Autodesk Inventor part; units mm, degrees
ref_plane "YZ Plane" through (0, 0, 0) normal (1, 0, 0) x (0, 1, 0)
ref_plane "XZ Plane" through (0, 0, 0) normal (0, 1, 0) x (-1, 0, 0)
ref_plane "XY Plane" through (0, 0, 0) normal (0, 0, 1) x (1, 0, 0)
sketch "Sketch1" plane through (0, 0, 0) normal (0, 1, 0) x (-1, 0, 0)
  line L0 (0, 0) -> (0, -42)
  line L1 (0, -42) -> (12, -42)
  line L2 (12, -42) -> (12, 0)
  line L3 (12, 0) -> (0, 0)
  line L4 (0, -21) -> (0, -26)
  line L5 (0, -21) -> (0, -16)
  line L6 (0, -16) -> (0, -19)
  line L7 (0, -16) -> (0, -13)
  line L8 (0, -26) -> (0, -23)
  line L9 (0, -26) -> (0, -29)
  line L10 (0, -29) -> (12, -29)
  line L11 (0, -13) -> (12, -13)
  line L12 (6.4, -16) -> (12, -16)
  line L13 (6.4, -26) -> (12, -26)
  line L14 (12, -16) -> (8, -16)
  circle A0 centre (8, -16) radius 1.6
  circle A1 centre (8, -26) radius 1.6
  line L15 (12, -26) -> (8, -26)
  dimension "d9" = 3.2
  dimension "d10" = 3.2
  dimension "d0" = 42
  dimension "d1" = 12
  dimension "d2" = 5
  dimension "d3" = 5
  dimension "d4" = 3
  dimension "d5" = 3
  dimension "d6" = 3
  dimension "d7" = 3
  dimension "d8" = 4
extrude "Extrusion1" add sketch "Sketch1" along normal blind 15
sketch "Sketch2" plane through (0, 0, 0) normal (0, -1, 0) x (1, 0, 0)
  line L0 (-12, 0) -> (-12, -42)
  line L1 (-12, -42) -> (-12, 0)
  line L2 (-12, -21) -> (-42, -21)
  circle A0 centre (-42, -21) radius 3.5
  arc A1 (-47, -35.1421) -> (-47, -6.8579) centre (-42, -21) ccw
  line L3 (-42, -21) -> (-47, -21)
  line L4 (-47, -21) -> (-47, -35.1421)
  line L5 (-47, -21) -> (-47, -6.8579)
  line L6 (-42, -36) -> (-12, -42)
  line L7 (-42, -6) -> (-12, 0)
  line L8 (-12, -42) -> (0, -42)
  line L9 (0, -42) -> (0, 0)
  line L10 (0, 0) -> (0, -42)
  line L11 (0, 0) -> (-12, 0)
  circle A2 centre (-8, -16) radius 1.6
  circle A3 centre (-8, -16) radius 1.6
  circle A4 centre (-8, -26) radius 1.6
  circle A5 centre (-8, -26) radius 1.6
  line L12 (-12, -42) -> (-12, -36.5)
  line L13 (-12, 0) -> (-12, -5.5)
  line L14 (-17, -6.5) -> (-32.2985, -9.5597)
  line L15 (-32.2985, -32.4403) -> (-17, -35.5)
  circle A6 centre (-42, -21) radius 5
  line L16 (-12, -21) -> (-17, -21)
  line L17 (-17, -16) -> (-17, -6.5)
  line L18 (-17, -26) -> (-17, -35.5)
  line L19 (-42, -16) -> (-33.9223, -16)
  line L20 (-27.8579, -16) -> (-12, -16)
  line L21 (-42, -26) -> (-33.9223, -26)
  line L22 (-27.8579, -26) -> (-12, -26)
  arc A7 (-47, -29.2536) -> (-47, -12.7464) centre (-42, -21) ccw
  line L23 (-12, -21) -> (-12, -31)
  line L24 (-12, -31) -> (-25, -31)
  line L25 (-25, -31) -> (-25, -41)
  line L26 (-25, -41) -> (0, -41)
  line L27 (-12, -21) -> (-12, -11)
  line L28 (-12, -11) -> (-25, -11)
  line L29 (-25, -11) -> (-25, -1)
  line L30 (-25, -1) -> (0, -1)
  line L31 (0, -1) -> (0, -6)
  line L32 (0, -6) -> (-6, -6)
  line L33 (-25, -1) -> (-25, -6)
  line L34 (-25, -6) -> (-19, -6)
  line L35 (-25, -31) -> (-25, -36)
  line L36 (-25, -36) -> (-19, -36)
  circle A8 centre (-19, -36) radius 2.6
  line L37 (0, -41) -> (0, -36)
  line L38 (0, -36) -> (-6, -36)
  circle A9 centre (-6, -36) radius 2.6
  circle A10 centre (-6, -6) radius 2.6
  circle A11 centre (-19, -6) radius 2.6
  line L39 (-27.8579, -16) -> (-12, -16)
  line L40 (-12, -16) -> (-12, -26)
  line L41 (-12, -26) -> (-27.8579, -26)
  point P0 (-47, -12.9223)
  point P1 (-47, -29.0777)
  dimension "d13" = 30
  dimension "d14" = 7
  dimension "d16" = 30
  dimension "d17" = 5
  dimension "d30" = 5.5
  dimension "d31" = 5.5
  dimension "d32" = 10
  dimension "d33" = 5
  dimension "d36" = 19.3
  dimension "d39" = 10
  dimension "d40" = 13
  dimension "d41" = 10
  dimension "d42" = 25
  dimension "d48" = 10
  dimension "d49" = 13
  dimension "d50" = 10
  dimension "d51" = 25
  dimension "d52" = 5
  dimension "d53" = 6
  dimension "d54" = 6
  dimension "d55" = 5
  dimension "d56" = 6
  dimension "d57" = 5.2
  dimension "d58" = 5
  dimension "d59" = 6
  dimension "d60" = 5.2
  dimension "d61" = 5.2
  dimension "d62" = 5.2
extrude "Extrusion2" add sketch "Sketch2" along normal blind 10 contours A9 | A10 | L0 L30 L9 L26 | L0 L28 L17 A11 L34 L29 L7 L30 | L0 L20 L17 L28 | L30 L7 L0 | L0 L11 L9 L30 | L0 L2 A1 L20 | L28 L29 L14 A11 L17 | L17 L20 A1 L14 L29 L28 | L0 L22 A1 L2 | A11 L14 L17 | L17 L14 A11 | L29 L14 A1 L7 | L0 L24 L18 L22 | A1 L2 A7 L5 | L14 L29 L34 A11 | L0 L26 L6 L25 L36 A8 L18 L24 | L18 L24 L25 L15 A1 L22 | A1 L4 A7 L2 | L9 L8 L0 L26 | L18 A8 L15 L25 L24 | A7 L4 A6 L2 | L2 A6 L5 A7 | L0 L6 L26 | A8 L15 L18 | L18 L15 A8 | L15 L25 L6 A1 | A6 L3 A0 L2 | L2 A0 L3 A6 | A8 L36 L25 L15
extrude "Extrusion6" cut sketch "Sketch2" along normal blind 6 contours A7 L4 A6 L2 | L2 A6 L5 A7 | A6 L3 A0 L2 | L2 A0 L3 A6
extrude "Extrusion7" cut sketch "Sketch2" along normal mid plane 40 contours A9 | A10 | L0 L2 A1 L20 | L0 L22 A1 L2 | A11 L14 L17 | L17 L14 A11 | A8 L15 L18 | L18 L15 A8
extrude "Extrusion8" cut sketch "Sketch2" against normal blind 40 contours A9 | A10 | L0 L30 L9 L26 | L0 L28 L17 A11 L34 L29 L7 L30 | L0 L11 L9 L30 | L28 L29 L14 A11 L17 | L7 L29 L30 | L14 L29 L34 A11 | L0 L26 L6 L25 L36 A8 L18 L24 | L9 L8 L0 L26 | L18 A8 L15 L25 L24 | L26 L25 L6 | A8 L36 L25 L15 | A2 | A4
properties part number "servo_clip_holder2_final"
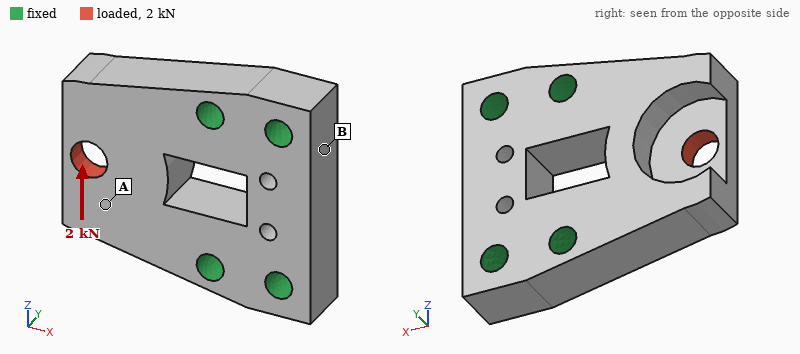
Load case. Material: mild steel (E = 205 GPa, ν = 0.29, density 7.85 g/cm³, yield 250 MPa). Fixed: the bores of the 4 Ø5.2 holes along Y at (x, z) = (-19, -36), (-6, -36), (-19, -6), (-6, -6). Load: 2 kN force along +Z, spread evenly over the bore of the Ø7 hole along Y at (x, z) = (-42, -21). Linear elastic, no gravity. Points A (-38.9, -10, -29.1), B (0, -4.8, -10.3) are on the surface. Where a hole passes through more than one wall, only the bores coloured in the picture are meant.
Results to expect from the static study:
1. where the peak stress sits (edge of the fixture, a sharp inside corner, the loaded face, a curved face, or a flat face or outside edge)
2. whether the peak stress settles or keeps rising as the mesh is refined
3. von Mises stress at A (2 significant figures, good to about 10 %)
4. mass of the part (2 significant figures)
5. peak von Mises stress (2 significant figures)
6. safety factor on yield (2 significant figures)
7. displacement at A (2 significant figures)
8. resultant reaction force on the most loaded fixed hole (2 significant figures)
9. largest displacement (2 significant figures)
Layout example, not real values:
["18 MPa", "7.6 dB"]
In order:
["the loaded face", "settles", "23 MPa", "100 g", "85 MPa", "2.9", "3.9 µm", "1.7 kN", "7.1 µm"]
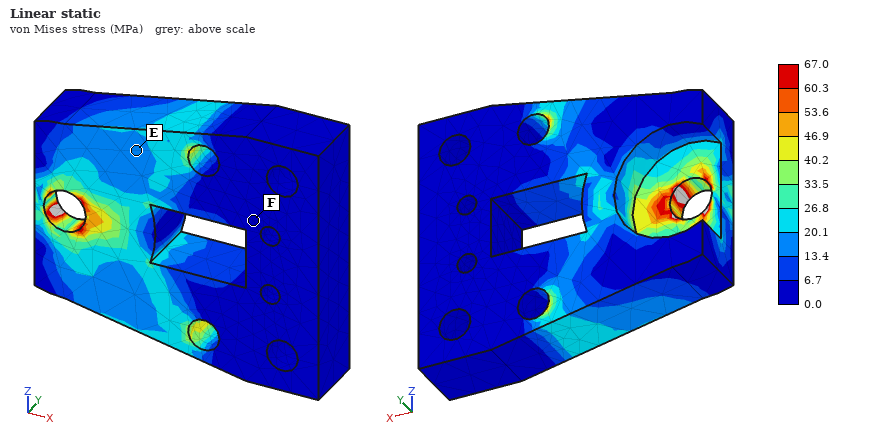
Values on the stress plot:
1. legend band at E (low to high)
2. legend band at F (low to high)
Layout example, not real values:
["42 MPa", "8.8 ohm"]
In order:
["13.4 to 20.1 MPa", "0.0 to 6.7 MPa"]
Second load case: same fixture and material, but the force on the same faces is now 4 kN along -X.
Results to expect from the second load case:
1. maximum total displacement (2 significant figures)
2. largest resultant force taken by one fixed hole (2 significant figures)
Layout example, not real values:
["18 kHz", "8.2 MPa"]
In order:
["15 µm", "1.8 kN"]
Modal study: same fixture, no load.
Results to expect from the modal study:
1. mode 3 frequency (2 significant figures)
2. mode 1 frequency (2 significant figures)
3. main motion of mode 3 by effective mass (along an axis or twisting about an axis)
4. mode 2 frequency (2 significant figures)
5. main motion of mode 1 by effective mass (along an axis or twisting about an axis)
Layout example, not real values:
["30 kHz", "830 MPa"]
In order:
["23 kHz", "11 kHz", "along Z", "16 kHz", "along Y"]
